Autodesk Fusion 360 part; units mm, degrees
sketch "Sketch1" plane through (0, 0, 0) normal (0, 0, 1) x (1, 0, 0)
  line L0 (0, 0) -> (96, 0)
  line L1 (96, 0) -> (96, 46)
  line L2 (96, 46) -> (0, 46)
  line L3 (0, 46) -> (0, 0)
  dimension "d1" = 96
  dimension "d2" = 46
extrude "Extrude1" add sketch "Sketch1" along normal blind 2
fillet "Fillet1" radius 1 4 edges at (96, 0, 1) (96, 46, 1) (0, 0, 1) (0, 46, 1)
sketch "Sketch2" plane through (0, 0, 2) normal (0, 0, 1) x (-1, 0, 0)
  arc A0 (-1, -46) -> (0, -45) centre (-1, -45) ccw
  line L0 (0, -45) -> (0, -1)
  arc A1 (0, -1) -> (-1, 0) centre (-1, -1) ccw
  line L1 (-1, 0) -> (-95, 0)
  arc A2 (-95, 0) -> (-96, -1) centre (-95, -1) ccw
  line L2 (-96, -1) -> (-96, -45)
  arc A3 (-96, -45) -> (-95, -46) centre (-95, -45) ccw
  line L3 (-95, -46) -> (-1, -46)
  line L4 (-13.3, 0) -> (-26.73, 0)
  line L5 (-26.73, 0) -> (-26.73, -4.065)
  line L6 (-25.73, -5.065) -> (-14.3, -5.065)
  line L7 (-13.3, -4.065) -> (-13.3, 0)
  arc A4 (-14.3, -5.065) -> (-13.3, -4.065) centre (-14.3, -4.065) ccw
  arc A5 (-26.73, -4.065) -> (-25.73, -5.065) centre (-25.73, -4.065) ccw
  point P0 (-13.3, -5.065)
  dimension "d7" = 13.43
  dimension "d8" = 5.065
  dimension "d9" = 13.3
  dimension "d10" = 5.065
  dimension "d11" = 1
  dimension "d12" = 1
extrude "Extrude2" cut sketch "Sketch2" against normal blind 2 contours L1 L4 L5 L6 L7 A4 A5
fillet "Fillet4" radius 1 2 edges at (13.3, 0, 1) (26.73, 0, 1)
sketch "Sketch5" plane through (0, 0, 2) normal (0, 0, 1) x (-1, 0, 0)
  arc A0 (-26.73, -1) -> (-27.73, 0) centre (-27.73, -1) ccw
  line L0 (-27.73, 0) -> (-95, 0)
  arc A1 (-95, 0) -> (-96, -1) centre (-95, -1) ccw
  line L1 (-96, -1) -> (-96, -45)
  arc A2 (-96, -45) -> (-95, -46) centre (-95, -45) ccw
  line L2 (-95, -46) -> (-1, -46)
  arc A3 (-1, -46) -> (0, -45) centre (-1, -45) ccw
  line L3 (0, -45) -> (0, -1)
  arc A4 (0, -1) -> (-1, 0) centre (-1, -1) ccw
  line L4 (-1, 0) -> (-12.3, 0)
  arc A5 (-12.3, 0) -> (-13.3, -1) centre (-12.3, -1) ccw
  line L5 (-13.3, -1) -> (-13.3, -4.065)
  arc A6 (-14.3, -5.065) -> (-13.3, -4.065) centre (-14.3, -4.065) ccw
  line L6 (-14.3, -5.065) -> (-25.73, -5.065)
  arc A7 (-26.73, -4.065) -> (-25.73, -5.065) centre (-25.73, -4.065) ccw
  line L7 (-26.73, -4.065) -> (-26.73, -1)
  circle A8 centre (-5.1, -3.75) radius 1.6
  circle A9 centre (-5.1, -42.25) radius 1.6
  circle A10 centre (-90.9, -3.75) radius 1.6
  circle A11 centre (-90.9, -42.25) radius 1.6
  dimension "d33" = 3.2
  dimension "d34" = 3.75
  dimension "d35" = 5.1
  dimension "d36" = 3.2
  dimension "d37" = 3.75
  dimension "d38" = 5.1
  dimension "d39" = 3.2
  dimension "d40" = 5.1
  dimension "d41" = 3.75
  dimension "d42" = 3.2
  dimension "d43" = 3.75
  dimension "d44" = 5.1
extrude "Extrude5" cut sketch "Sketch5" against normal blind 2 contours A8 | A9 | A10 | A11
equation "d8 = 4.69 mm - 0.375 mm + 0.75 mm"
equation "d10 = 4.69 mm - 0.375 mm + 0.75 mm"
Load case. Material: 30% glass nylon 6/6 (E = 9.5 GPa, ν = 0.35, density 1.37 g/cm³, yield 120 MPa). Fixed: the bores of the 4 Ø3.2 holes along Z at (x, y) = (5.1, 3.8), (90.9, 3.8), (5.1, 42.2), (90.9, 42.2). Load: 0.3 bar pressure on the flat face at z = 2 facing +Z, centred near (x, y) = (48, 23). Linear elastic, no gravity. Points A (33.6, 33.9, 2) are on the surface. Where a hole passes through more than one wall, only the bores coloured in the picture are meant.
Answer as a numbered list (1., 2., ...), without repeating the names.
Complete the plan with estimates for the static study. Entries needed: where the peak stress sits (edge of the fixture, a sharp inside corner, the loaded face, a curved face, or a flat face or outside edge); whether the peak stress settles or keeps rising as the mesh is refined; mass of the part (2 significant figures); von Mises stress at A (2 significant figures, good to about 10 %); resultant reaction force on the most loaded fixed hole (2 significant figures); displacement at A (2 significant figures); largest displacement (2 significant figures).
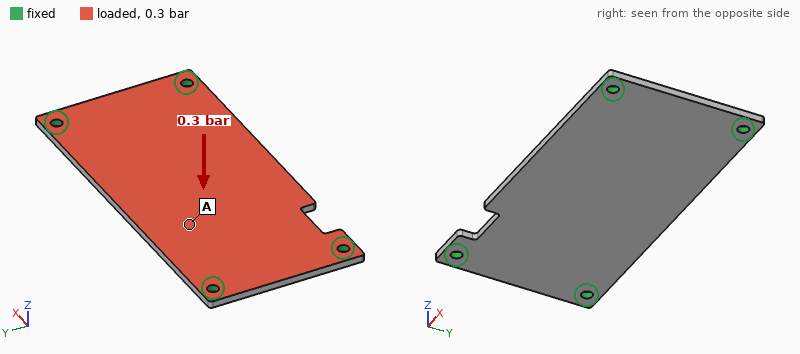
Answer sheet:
1. edge of the fixture
2. keeps rising
3. 12 g
4. 10 MPa
5. 33 N
6. 0.65 mm
7. 0.87 mm
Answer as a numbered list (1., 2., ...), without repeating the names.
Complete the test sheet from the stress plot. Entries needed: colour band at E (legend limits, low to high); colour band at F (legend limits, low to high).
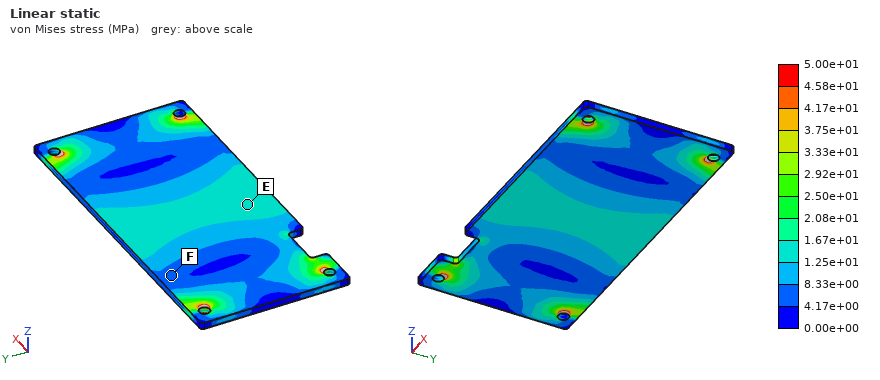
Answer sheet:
1. 1.25e+01 to 1.67e+01 MPa
2. 4.17e+00 to 8.33e+00 MPa
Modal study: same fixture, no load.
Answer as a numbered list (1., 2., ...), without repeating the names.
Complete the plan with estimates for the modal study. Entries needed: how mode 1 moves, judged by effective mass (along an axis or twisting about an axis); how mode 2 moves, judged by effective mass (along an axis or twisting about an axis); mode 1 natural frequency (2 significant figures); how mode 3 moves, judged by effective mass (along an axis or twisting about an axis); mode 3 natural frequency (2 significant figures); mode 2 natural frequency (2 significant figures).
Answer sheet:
1. along Z
2. twisting about X
3. 660 Hz
4. twisting about Y
5. 1800 Hz
6. 1100 Hz
